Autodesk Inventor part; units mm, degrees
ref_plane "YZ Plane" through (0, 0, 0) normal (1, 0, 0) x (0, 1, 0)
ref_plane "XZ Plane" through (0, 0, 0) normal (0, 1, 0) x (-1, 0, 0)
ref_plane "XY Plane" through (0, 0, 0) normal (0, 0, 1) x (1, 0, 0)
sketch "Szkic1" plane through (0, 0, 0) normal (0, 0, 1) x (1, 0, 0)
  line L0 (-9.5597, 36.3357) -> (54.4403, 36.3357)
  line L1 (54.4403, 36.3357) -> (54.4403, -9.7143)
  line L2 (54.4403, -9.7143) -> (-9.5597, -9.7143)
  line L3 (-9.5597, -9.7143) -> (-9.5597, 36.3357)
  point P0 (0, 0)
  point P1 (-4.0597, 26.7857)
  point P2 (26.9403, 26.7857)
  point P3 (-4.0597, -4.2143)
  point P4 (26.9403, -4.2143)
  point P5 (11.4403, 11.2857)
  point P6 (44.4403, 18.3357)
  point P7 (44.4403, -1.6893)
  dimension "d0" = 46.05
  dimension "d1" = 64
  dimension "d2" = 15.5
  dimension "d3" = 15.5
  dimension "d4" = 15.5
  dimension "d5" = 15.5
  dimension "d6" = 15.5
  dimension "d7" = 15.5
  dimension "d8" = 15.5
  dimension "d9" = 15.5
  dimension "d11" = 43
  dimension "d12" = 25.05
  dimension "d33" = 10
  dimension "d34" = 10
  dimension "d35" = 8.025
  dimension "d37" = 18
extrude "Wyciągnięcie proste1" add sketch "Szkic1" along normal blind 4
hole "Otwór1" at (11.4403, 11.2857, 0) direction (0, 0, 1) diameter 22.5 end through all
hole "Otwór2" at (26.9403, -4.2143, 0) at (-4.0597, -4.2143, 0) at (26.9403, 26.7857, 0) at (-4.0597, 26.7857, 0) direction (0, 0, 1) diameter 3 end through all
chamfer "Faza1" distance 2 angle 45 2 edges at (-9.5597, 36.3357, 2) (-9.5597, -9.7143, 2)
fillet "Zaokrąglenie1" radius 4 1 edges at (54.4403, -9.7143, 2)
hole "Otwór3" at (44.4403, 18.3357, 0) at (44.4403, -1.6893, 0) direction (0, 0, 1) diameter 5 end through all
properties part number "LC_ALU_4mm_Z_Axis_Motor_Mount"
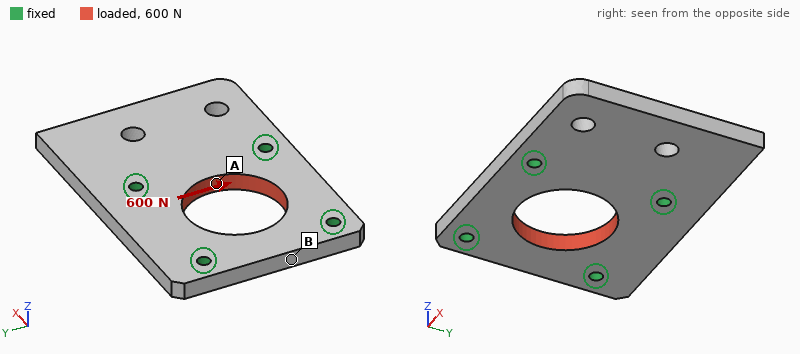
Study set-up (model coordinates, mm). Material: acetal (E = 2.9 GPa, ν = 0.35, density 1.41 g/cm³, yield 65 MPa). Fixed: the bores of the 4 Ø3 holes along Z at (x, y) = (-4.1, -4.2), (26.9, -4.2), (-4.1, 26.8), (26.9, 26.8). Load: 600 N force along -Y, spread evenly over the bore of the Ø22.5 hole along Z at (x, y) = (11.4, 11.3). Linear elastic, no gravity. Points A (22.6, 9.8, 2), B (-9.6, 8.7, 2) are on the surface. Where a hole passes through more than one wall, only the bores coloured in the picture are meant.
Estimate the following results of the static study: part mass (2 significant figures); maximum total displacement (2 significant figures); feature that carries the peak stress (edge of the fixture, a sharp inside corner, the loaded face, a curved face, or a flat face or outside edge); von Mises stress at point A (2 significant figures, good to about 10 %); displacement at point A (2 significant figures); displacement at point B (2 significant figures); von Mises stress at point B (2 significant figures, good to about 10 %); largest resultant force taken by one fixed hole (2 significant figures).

14 g
35 µm
edge of the fixture
3.7 MPa
15 µm
7.8 µm
1.3 MPa
160 N
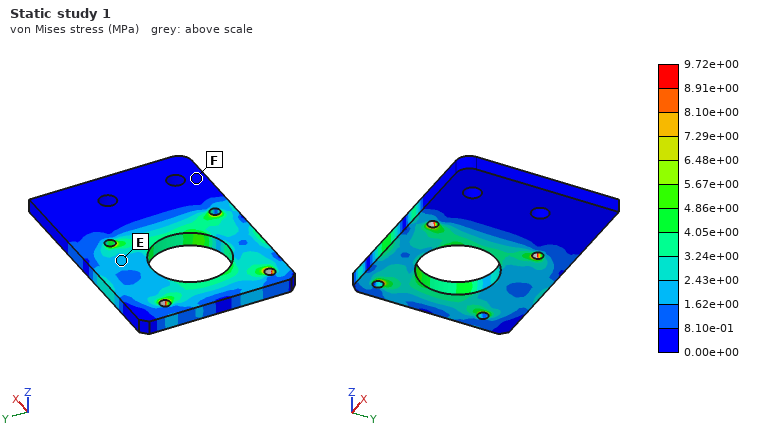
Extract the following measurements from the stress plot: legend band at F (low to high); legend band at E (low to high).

0.00e+00 to 8.10e-01 MPa
1.62e+00 to 2.43e+00 MPa
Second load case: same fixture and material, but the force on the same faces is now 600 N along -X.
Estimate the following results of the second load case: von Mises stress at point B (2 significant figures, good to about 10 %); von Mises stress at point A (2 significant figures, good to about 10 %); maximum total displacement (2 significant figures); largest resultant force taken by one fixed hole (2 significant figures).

4.4 MPa
2.0 MPa
37 µm
160 N
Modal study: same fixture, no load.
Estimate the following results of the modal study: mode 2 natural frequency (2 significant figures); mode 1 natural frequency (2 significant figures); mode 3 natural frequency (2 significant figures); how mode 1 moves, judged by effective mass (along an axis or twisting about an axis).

2000 Hz
1100 Hz
3800 Hz
along Z
